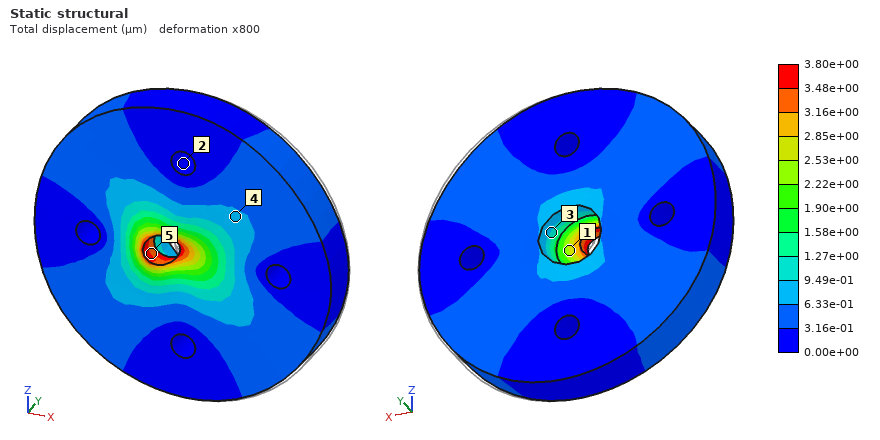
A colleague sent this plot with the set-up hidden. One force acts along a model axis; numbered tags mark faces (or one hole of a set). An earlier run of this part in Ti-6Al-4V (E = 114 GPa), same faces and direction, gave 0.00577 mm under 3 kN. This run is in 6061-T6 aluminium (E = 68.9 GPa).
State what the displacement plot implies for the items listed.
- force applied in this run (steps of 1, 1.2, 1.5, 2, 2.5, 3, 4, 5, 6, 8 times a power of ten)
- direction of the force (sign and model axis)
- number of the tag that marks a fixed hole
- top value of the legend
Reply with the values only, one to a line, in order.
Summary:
1.2 kN
-X
2
3.80e+00 µm
